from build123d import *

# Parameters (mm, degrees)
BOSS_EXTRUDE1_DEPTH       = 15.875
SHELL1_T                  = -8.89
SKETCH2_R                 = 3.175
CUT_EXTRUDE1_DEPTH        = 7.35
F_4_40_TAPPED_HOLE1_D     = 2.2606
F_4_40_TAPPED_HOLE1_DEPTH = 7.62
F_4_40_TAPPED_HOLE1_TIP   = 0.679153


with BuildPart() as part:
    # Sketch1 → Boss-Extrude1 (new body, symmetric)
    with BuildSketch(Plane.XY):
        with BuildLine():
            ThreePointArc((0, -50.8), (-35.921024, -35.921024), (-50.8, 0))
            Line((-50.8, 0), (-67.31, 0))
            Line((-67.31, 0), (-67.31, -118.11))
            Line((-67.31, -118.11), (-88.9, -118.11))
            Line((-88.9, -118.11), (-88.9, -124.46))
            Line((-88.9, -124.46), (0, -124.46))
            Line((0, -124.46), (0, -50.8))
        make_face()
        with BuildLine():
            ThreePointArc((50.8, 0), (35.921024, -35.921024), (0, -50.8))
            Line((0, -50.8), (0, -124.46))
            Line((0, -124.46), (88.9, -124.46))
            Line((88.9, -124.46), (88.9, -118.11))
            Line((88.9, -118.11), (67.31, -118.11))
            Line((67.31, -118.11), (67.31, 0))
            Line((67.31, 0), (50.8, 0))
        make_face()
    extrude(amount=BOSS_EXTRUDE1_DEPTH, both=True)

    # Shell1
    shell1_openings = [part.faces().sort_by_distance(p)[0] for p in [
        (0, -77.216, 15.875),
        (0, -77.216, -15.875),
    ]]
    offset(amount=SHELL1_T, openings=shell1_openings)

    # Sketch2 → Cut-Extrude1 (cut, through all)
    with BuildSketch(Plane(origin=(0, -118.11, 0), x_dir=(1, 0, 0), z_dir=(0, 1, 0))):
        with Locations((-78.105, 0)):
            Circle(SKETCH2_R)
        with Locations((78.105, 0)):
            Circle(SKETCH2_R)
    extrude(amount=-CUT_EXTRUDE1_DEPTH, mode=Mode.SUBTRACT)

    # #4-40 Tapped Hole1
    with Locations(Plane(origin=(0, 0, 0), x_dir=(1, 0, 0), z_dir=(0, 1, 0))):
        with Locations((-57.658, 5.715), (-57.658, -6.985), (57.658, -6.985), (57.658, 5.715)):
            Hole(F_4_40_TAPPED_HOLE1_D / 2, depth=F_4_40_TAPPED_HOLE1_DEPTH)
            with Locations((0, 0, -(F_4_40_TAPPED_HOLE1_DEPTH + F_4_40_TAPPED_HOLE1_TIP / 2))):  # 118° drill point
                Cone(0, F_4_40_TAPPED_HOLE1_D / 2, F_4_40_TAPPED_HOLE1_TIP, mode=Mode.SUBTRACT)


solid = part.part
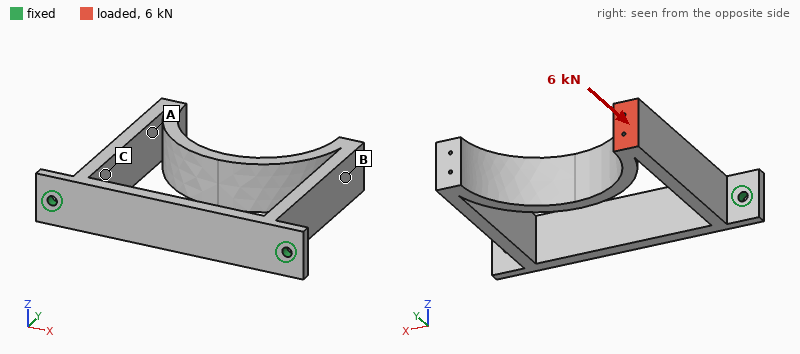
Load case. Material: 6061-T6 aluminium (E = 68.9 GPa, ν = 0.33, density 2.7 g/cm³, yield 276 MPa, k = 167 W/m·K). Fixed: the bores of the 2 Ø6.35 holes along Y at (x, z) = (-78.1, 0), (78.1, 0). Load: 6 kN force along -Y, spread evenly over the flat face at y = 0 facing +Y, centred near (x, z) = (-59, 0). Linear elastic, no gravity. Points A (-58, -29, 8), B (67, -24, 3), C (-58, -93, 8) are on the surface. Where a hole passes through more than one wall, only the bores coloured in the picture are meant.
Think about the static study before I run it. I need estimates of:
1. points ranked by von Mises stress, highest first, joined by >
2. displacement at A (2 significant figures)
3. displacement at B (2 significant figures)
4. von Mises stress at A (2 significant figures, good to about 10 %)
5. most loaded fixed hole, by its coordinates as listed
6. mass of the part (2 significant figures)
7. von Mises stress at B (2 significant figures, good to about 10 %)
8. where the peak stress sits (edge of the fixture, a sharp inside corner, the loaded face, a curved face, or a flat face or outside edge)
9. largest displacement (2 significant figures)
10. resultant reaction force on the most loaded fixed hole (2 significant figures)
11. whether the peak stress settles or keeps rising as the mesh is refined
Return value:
A > B > C
0.27 mm
0.087 mm
39 MPa
(-78.1, 0)
430 g
20 MPa
edge of the fixture
0.40 mm
5.6 kN
keeps rising
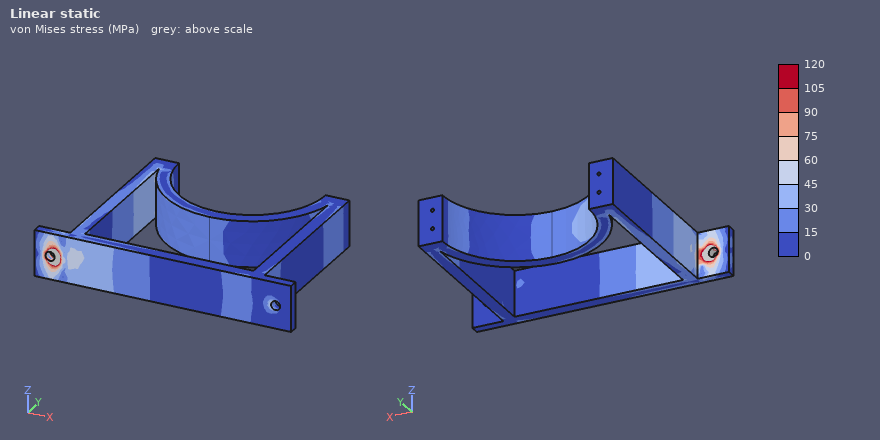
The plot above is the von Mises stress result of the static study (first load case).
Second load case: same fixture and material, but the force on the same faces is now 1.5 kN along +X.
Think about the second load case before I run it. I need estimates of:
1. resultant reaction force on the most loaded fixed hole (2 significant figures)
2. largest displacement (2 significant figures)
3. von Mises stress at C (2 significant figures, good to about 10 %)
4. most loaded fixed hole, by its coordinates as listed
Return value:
1.4 kN
1.9 mm
79 MPa
(78.1, 0)
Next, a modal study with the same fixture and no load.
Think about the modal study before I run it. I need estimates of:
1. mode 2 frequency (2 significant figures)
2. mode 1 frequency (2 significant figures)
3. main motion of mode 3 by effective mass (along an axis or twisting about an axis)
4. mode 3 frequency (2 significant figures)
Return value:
400 Hz
390 Hz
twisting about Y
660 Hz
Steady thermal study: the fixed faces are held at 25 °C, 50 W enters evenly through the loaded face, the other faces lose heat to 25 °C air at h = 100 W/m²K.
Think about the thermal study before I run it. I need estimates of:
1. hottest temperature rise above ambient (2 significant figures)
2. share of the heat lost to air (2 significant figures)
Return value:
42 K
84 %
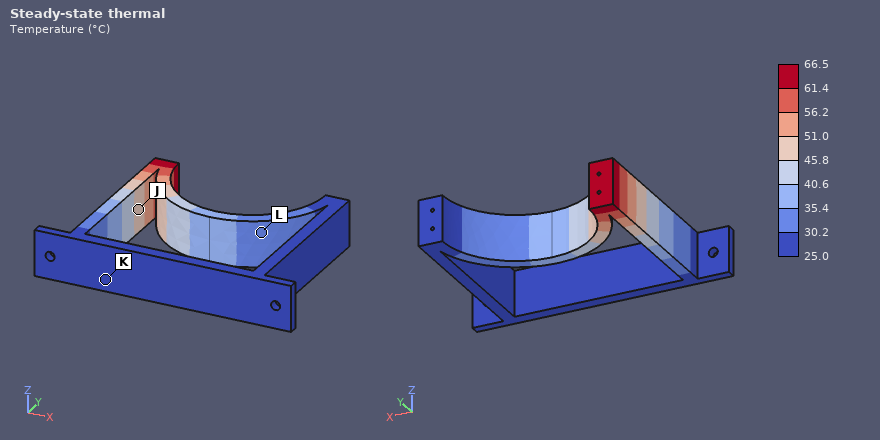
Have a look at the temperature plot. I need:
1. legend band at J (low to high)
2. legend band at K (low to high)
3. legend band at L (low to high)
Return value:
45.8 to 51.0 °C
25.0 to 30.2 °C
30.2 to 35.4 °C
